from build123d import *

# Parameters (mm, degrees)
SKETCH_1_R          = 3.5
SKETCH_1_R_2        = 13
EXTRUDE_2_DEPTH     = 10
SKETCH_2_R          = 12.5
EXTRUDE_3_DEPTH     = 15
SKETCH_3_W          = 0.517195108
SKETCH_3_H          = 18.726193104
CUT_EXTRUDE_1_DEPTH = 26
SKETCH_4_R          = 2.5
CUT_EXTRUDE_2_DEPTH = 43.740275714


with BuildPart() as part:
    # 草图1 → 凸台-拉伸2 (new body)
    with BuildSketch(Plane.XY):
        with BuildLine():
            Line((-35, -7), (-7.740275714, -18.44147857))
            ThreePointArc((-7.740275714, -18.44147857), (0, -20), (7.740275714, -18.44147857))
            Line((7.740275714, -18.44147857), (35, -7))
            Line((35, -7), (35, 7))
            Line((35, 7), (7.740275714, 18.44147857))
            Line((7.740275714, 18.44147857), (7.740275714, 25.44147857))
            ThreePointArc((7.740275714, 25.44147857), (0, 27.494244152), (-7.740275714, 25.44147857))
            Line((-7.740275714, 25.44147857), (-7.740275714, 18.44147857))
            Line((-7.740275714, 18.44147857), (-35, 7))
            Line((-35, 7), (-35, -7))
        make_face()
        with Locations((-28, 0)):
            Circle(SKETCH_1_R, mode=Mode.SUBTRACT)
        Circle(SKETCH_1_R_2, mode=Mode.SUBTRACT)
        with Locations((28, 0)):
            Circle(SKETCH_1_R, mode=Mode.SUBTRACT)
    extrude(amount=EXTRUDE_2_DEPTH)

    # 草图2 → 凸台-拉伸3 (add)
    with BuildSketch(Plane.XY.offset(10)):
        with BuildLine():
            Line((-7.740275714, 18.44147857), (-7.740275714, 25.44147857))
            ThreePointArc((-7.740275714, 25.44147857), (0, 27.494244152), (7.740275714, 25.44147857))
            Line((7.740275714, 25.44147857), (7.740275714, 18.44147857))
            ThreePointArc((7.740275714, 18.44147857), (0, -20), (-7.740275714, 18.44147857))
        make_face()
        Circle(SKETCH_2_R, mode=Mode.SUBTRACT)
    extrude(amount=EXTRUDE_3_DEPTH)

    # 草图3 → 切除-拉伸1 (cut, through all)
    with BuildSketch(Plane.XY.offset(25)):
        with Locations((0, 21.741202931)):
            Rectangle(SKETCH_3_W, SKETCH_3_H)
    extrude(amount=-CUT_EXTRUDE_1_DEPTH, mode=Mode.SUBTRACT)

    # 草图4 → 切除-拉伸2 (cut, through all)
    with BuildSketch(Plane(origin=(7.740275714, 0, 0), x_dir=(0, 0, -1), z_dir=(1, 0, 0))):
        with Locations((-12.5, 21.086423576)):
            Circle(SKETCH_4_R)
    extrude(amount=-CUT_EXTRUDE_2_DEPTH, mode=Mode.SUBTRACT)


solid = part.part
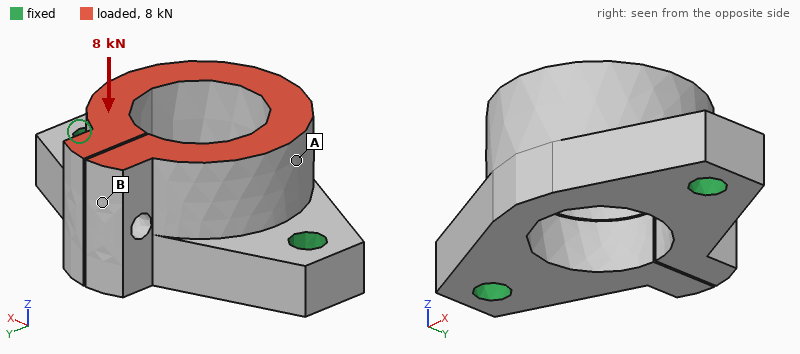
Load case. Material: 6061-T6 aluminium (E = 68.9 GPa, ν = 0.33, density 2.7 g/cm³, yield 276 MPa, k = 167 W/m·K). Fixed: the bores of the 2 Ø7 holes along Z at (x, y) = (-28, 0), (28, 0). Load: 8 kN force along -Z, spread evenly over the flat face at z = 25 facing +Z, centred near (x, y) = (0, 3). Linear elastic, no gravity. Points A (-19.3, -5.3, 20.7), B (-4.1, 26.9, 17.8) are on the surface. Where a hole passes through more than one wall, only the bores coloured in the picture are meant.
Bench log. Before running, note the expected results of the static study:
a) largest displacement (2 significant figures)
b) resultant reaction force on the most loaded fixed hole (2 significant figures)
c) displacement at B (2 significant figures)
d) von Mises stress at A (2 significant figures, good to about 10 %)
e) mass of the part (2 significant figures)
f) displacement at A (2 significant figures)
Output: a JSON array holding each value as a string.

["0.14 mm", "4.1 kN", "0.11 mm", "42 MPa", "75 g", "0.033 mm"]
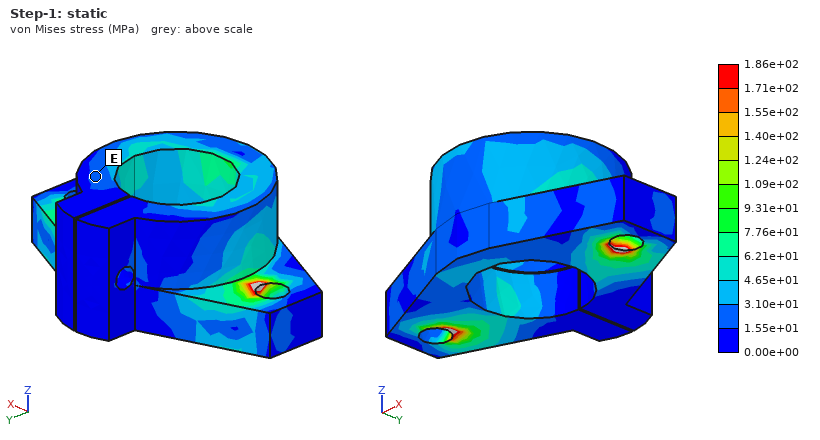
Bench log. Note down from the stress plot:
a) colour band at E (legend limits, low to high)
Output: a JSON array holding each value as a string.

["1.55e+01 to 3.10e+01 MPa"]
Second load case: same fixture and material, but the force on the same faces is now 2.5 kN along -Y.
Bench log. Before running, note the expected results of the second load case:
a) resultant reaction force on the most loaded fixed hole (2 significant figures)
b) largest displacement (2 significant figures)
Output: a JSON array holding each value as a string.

["1.4 kN", "79 µm"]
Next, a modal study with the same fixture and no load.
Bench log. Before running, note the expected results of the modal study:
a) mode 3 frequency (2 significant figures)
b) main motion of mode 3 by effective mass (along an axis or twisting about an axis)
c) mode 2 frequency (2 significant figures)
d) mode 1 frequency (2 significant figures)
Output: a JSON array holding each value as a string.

["6300 Hz", "along Y", "5700 Hz", "5700 Hz"]
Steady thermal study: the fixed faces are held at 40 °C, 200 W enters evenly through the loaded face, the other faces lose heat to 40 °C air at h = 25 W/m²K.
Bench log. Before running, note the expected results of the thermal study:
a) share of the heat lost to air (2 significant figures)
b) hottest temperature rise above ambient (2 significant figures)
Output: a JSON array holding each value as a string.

["4.0 %", "67 K"]
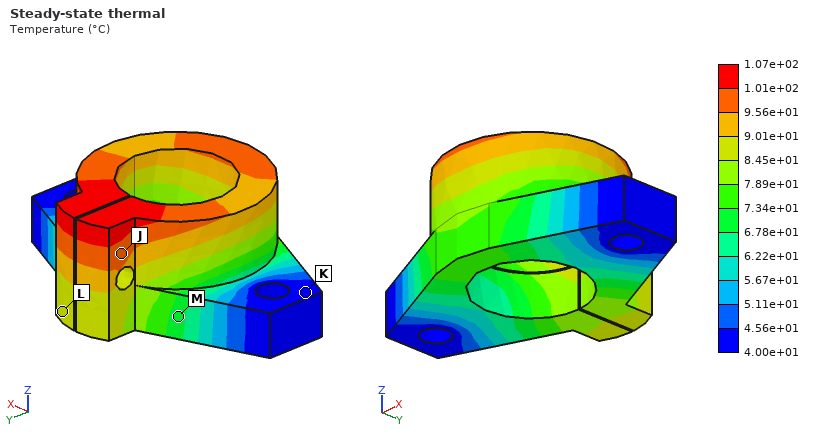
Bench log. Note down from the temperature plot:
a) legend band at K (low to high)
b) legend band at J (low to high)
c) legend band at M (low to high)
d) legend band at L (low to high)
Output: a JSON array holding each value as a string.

["4.00e+01 to 4.56e+01 °C", "9.56e+01 to 1.01e+02 °C", "6.78e+01 to 7.34e+01 °C", "8.45e+01 to 9.01e+01 °C"]
